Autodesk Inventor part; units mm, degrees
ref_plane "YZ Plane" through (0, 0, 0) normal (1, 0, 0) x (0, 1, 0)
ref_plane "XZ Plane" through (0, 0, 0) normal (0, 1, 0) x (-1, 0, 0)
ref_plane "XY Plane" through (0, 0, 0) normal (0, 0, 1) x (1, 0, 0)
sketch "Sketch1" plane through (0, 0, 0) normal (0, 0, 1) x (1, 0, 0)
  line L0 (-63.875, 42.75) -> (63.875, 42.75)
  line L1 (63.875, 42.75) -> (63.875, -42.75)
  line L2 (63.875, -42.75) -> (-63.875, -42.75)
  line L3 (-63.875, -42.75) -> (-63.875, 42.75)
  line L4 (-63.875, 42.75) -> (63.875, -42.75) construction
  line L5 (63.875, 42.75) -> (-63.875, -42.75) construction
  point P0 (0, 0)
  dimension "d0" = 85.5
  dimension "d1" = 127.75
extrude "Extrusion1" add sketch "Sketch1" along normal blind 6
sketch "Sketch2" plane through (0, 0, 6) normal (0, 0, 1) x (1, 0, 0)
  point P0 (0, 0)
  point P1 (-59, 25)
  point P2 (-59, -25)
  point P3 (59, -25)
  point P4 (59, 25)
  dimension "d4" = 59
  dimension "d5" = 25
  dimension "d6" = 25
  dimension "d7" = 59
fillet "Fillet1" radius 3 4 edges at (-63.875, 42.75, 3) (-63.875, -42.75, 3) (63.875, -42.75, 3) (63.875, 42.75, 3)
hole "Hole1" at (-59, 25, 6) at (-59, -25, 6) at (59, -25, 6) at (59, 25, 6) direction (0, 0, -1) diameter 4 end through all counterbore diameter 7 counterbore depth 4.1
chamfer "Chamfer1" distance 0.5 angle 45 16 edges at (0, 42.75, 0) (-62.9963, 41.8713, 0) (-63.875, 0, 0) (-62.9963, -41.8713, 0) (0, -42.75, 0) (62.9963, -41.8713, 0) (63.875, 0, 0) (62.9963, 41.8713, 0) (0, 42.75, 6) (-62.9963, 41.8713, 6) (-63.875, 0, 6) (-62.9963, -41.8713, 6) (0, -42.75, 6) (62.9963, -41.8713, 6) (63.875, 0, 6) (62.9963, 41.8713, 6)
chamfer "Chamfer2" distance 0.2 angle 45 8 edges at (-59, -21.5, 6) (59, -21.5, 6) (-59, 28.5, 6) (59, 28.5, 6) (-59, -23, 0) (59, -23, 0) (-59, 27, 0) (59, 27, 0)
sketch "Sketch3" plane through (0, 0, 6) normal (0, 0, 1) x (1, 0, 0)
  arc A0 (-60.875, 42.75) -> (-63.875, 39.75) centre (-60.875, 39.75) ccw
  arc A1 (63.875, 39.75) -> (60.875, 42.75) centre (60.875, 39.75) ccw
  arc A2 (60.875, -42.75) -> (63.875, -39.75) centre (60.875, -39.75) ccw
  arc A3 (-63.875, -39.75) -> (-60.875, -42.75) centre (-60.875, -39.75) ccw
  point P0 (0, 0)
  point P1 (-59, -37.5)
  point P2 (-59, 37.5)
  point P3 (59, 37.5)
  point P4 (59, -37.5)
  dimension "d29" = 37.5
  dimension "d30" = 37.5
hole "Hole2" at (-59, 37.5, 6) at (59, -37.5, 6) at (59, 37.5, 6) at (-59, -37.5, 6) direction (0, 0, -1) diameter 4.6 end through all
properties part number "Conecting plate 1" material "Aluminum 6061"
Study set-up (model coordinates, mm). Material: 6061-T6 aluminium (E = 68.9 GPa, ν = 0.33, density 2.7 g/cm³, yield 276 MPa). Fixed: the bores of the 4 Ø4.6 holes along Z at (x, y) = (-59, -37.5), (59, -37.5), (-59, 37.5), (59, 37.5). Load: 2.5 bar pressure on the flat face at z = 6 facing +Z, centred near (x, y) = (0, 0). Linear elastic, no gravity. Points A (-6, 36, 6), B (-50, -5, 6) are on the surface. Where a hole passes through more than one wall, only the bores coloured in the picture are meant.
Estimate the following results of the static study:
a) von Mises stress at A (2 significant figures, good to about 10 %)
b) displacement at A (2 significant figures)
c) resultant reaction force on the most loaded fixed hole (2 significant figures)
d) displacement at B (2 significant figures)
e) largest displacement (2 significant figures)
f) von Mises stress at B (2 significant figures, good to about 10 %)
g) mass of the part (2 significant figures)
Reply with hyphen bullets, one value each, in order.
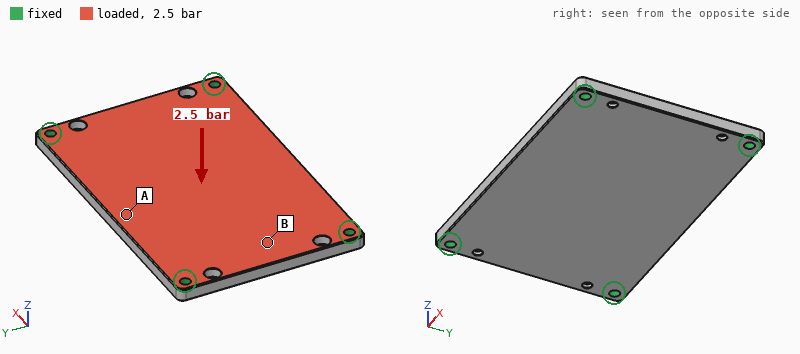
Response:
- 33 MPa
- 0.16 mm
- 660 N
- 0.059 mm
- 0.18 mm
- 16 MPa
- 170 g
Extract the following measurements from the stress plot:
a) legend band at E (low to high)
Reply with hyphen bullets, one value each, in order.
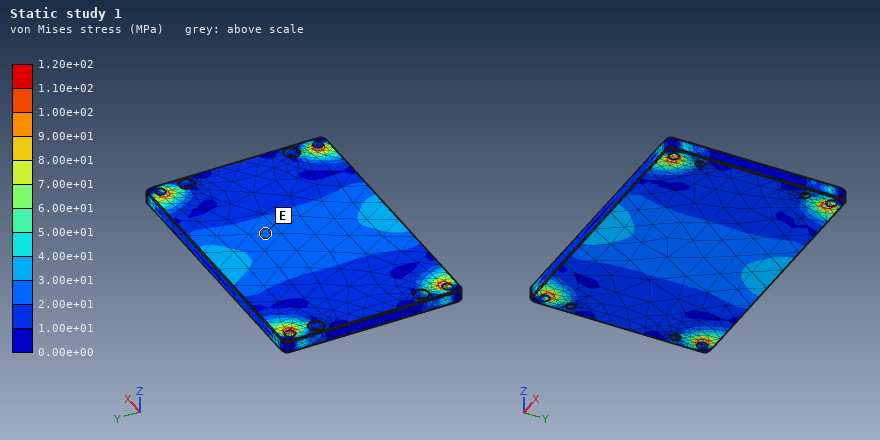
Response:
- 2.00e+01 to 3.00e+01 MPa
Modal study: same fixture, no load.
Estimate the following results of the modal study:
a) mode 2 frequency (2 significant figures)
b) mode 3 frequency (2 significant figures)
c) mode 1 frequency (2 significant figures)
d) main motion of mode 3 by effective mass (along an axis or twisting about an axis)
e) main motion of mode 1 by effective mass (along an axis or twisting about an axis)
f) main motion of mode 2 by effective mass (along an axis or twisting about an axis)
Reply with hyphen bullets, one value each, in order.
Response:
- 2900 Hz
- 4300 Hz
- 1700 Hz
- twisting about Y
- along Z
- twisting about X
